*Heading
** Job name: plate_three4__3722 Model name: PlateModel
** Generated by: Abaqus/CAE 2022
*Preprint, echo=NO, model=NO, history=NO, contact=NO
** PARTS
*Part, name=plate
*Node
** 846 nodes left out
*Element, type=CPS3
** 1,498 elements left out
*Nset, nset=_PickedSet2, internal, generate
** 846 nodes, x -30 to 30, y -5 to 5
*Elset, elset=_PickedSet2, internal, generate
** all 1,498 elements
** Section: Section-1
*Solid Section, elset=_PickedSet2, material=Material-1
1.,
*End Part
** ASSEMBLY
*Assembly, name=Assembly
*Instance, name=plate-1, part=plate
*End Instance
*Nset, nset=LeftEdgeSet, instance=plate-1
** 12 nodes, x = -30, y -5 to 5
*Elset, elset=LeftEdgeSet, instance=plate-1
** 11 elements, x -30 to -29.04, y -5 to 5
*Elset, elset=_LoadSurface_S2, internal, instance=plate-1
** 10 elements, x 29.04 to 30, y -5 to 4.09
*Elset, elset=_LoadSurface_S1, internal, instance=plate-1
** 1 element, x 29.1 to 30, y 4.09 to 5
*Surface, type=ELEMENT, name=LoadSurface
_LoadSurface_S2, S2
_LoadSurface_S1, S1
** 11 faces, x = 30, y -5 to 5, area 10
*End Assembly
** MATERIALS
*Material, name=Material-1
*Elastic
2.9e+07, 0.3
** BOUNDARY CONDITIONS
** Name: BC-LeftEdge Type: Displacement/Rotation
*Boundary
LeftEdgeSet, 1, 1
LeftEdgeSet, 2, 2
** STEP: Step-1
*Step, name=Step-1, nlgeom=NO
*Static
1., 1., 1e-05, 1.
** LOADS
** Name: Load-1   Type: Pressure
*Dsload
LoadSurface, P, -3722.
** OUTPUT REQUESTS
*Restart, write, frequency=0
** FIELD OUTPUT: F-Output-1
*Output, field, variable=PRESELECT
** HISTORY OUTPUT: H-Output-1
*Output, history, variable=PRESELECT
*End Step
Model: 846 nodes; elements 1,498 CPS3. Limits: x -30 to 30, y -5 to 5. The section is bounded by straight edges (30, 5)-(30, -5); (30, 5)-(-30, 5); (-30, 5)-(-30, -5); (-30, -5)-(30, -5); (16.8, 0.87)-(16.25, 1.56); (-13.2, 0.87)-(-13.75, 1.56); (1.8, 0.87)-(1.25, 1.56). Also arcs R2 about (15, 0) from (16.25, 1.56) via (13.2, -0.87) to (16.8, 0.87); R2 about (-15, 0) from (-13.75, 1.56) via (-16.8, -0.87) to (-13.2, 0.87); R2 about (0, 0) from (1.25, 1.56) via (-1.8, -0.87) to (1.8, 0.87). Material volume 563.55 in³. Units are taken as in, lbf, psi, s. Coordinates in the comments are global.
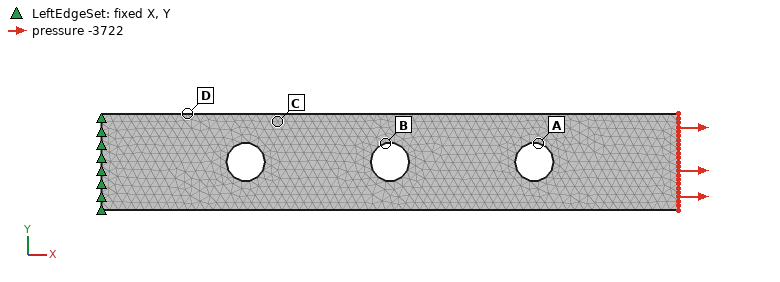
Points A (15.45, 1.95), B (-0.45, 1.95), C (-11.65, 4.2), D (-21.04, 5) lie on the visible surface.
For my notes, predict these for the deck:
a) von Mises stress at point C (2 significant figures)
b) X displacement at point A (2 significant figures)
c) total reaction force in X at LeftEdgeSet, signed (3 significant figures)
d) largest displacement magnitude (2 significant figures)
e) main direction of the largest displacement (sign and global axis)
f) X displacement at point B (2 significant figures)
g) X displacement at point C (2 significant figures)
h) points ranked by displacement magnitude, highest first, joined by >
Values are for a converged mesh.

5200 psi
0.0074 in
-37200 lbf
0.0094 in
+X
0.0045 in
0.0027 in
A > B > C > D
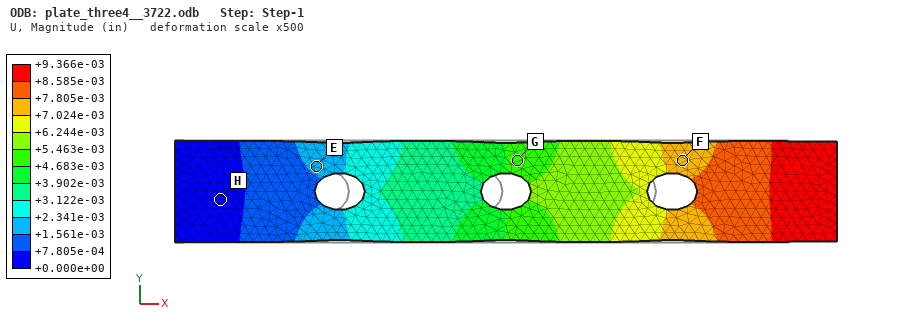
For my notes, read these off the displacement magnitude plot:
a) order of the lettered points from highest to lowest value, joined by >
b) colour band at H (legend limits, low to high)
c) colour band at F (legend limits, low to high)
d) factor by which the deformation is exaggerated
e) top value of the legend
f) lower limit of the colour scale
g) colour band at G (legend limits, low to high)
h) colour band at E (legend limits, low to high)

F > G > E > H
+0.000e+00 to +7.805e-04 in
+7.024e-03 to +7.805e-03 in
500
+9.366e-03 in
+0.000e+00 in
+4.683e-03 to +5.463e-03 in
+1.561e-03 to +2.341e-03 in
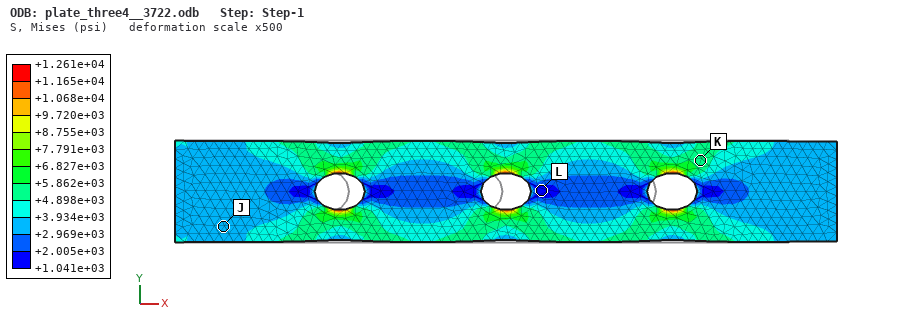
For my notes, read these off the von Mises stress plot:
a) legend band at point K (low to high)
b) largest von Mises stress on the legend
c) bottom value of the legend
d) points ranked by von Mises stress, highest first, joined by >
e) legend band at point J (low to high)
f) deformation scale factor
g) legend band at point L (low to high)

+4.898e+03 to +5.862e+03 psi
+1.261e+04 psi
+1.041e+03 psi
K > J > L
+2.969e+03 to +3.934e+03 psi
500
+1.041e+03 to +2.005e+03 psi
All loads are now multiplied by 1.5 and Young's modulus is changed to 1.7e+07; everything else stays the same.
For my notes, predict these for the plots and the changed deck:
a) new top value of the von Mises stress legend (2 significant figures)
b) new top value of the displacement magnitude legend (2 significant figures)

19000 psi
0.024 in
